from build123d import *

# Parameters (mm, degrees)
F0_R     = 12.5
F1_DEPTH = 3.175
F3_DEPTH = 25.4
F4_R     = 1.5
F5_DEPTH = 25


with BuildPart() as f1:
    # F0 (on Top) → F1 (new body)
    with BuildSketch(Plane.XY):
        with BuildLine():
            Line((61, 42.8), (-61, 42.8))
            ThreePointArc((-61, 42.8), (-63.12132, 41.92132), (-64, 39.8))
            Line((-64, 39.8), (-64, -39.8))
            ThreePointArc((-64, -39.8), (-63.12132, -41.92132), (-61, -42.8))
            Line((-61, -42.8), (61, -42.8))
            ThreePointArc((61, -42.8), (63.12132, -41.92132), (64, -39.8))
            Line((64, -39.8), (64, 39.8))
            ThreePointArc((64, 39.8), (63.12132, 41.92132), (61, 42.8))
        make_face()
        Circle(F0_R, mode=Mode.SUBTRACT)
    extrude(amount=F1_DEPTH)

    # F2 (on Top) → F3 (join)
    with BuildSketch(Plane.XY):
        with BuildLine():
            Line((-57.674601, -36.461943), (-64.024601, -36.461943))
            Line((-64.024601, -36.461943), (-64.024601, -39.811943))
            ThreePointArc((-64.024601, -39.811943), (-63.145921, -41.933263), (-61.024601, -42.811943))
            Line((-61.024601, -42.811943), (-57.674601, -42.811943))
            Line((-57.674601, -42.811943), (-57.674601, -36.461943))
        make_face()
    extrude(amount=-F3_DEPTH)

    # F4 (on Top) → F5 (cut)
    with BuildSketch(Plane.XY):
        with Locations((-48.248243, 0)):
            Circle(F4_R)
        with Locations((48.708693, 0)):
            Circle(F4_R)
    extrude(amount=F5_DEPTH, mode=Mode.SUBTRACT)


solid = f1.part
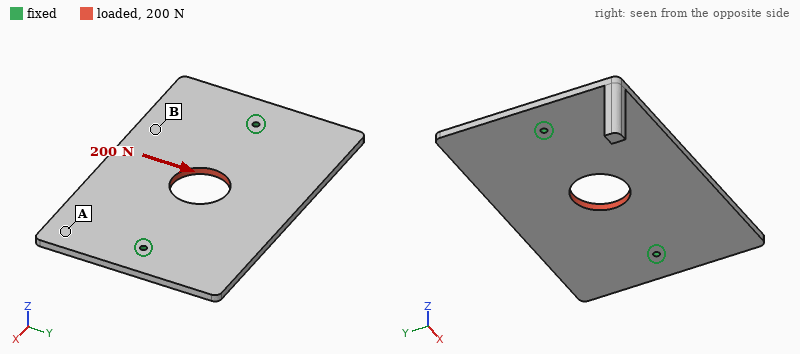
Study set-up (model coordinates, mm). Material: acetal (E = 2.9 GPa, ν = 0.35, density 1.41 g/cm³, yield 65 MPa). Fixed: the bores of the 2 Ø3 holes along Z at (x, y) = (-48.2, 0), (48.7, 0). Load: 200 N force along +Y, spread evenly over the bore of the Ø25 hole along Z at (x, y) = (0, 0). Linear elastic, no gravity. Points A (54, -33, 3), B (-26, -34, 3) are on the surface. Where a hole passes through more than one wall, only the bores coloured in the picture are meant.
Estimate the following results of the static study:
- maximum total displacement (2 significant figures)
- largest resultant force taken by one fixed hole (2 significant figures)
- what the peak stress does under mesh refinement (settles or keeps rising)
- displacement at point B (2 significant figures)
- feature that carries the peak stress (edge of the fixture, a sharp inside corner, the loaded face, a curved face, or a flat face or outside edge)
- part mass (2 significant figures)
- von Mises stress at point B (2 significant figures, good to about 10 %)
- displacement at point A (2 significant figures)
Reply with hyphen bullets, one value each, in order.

- 32 µm
- 100 N
- keeps rising
- 20 µm
- edge of the fixture
- 48 g
- 0.64 MPa
- 9.6 µm
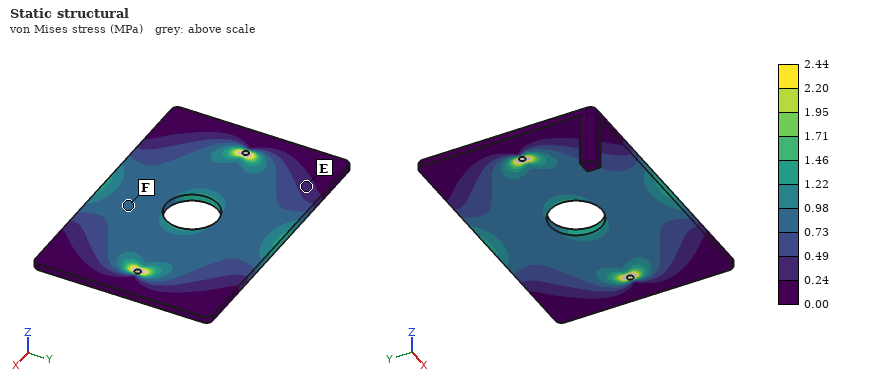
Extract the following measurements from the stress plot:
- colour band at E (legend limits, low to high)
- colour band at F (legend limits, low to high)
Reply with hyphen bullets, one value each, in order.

- 0.24 to 0.49 MPa
- 0.73 to 0.98 MPa
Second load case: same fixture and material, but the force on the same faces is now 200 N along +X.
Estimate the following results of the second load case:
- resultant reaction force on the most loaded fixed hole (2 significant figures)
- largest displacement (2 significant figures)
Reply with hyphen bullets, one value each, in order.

- 100 N
- 18 µm
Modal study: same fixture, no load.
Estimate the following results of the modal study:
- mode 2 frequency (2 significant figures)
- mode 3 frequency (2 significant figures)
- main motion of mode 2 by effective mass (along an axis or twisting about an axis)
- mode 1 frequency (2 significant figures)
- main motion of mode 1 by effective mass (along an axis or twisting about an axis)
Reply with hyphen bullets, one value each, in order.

- 290 Hz
- 340 Hz
- along Z
- 210 Hz
- twisting about X
